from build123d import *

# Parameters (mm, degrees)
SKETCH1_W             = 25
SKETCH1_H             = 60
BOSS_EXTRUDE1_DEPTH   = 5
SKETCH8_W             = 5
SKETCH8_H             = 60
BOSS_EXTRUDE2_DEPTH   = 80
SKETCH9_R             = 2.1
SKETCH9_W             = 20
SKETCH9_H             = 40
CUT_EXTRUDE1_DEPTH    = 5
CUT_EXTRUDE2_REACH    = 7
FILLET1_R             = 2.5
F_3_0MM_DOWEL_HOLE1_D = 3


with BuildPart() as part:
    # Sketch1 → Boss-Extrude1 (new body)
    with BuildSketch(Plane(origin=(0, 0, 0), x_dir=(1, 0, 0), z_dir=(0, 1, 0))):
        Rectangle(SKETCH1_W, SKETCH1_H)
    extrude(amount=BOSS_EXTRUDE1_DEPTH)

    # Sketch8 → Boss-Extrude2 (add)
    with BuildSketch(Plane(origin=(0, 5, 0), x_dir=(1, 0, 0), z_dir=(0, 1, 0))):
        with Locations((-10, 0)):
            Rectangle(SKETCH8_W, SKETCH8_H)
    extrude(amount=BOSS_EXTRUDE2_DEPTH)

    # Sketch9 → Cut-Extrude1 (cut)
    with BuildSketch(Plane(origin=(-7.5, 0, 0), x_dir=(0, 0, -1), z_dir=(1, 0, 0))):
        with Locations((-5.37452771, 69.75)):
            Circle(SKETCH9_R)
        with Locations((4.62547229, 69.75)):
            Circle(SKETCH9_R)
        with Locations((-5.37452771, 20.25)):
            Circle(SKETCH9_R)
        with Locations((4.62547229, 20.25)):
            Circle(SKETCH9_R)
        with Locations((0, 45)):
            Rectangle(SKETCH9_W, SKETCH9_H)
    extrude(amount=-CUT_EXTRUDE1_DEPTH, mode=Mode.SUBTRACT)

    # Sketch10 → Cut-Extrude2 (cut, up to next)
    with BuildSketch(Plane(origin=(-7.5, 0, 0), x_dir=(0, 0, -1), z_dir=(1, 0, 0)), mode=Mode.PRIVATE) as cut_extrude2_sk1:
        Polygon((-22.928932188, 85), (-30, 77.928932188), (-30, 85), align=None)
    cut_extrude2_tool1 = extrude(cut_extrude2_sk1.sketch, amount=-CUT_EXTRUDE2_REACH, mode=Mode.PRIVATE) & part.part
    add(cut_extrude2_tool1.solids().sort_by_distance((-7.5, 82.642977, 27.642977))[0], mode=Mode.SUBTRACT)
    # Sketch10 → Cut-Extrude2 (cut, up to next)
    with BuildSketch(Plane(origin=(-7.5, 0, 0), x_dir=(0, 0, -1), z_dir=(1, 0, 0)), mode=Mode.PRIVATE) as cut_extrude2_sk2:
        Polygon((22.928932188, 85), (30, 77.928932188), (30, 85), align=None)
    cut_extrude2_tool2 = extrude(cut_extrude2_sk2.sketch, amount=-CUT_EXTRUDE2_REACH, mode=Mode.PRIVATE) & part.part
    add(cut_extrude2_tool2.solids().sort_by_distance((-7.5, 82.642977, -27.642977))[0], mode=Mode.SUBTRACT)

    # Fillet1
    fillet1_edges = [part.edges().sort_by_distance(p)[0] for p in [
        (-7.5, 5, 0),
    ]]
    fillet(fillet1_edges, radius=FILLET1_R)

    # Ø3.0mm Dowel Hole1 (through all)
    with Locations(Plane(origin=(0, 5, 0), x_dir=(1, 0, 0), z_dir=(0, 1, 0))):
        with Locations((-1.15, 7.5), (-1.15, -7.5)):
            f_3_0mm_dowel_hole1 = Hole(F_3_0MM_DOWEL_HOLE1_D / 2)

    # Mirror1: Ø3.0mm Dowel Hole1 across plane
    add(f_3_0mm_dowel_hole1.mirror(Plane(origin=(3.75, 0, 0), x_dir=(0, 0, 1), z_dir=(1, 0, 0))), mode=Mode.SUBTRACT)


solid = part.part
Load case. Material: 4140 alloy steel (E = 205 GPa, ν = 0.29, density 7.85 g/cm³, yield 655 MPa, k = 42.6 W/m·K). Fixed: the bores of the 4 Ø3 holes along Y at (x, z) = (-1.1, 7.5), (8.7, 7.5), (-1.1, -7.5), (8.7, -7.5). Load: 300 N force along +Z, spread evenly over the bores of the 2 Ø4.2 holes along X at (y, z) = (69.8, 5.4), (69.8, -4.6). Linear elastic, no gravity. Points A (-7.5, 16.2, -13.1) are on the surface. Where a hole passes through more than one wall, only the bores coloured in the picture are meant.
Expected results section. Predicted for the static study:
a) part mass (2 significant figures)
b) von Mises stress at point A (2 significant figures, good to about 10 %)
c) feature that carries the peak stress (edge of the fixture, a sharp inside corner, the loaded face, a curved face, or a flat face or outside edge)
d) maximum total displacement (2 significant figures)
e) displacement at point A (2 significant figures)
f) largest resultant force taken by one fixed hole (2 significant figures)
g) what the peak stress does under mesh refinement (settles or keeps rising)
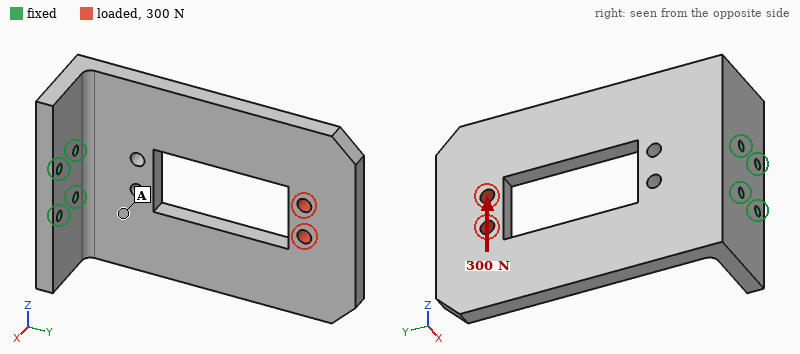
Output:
210 g
8.8 MPa
edge of the fixture
50 µm
9.7 µm
990 N
keeps rising
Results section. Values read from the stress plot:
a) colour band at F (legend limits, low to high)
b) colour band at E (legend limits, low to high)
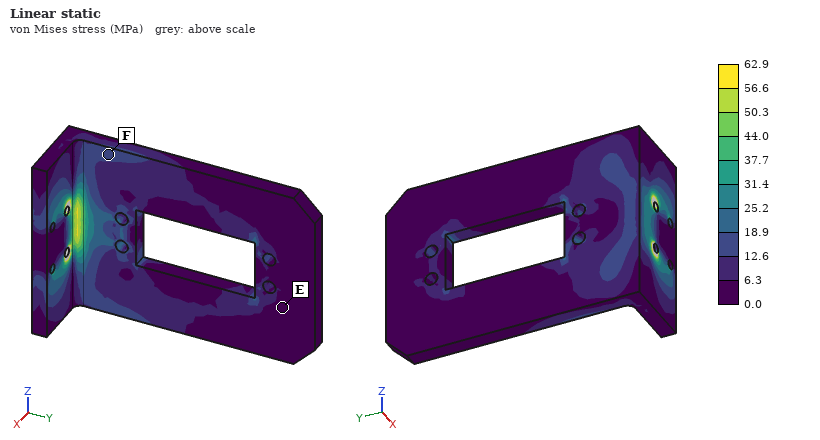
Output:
12.6 to 18.9 MPa
0.0 to 6.3 MPa
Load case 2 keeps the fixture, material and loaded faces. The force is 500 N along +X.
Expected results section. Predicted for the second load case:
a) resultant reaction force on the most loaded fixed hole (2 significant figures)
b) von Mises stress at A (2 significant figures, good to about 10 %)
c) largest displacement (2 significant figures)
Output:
810 N
110 MPa
0.82 mm
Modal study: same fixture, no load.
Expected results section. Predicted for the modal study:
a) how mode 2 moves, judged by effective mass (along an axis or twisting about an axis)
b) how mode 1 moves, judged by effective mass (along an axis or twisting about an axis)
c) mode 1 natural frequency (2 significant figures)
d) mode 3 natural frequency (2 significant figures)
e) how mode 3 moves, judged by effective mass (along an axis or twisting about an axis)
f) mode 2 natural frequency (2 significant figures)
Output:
along Z
along X
530 Hz
1700 Hz
along Z
1400 Hz
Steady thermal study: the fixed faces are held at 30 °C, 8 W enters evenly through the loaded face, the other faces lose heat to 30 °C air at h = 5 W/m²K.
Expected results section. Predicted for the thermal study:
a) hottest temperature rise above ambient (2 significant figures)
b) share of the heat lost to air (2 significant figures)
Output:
70 K
22 %
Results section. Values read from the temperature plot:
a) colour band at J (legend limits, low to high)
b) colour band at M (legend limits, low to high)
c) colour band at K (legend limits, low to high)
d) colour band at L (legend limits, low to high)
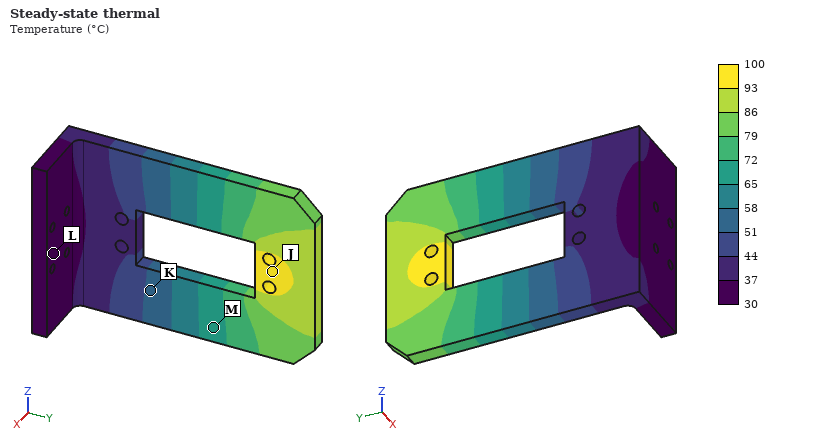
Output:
93 to 100 °C
65 to 72 °C
51 to 58 °C
30 to 37 °C
